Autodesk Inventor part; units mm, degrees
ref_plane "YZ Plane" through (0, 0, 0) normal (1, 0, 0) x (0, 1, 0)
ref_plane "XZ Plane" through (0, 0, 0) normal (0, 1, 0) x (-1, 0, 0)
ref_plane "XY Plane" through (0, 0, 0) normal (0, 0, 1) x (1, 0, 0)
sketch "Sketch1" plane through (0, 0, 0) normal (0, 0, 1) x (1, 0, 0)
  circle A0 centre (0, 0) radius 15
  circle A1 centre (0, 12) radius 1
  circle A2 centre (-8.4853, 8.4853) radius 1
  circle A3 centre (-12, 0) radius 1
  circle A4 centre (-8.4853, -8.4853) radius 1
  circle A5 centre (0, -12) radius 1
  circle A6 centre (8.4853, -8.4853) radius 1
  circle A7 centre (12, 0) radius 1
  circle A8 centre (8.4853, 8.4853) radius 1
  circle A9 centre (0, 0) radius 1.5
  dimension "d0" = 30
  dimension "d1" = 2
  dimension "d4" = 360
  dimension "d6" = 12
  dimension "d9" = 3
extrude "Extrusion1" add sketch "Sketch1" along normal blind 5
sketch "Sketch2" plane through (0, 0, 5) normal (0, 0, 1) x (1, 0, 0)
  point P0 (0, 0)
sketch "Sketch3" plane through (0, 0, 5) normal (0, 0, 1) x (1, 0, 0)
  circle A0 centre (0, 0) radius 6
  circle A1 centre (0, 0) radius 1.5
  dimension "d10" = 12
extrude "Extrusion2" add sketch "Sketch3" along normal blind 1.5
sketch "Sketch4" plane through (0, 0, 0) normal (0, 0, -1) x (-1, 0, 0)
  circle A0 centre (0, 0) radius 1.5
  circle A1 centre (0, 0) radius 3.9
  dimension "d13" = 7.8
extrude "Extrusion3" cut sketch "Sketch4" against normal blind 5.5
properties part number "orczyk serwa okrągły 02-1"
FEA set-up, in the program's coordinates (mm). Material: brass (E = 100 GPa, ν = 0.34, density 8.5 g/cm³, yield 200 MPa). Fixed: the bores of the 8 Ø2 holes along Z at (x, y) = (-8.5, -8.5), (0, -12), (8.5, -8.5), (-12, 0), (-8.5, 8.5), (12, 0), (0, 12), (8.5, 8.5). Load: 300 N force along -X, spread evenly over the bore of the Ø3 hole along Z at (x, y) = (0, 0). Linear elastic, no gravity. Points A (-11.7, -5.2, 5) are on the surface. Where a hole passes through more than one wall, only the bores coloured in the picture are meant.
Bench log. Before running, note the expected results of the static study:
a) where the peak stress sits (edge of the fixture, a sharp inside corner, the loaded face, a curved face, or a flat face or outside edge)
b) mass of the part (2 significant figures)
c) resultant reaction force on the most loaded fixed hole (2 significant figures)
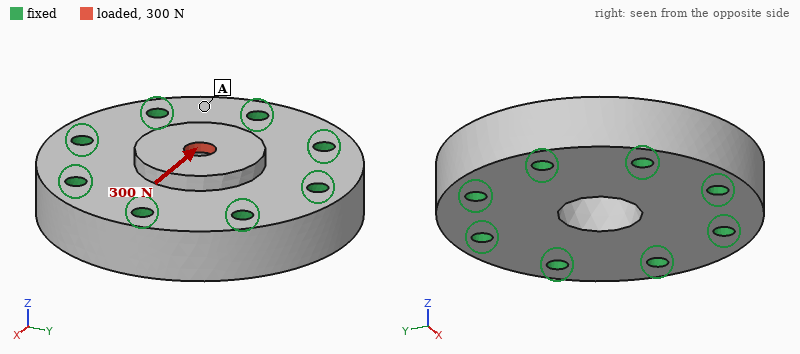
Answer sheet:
the loaded face
28 g
67 N
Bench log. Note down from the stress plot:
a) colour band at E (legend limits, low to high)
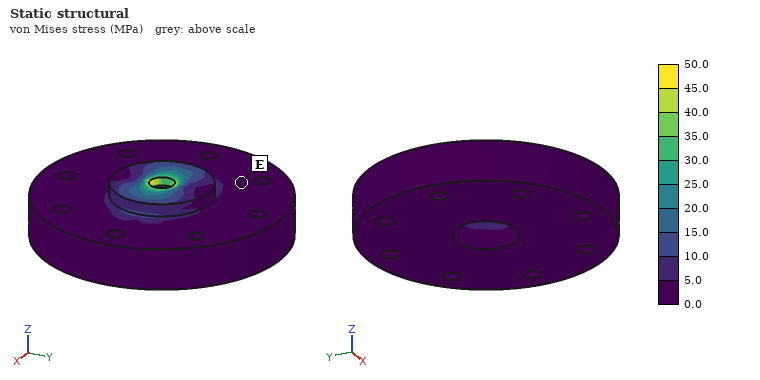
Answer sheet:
0.0 to 5.0 MPa
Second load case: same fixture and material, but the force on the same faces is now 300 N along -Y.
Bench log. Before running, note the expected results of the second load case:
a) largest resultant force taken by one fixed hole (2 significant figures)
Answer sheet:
67 N
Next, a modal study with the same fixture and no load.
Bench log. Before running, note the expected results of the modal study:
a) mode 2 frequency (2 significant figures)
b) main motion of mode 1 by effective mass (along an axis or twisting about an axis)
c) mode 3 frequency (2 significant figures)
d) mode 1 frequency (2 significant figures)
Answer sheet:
62 kHz
along Z
62 kHz
44 kHz
